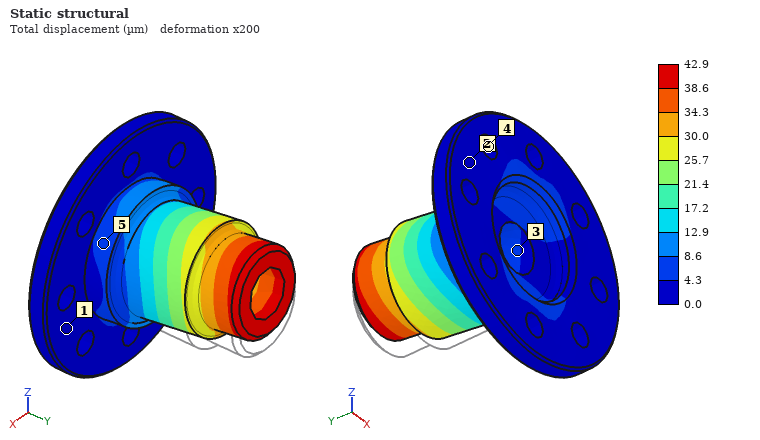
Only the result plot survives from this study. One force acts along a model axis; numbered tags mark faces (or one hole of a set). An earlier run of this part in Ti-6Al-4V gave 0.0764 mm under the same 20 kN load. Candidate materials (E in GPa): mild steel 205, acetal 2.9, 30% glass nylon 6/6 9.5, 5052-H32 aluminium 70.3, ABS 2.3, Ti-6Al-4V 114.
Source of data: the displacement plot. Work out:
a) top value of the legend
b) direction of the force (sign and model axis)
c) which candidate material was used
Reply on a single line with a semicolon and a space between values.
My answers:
42.9 µm; +Z; mild steel
